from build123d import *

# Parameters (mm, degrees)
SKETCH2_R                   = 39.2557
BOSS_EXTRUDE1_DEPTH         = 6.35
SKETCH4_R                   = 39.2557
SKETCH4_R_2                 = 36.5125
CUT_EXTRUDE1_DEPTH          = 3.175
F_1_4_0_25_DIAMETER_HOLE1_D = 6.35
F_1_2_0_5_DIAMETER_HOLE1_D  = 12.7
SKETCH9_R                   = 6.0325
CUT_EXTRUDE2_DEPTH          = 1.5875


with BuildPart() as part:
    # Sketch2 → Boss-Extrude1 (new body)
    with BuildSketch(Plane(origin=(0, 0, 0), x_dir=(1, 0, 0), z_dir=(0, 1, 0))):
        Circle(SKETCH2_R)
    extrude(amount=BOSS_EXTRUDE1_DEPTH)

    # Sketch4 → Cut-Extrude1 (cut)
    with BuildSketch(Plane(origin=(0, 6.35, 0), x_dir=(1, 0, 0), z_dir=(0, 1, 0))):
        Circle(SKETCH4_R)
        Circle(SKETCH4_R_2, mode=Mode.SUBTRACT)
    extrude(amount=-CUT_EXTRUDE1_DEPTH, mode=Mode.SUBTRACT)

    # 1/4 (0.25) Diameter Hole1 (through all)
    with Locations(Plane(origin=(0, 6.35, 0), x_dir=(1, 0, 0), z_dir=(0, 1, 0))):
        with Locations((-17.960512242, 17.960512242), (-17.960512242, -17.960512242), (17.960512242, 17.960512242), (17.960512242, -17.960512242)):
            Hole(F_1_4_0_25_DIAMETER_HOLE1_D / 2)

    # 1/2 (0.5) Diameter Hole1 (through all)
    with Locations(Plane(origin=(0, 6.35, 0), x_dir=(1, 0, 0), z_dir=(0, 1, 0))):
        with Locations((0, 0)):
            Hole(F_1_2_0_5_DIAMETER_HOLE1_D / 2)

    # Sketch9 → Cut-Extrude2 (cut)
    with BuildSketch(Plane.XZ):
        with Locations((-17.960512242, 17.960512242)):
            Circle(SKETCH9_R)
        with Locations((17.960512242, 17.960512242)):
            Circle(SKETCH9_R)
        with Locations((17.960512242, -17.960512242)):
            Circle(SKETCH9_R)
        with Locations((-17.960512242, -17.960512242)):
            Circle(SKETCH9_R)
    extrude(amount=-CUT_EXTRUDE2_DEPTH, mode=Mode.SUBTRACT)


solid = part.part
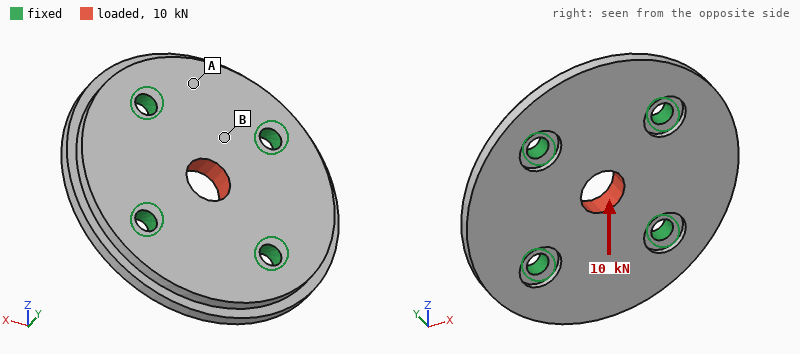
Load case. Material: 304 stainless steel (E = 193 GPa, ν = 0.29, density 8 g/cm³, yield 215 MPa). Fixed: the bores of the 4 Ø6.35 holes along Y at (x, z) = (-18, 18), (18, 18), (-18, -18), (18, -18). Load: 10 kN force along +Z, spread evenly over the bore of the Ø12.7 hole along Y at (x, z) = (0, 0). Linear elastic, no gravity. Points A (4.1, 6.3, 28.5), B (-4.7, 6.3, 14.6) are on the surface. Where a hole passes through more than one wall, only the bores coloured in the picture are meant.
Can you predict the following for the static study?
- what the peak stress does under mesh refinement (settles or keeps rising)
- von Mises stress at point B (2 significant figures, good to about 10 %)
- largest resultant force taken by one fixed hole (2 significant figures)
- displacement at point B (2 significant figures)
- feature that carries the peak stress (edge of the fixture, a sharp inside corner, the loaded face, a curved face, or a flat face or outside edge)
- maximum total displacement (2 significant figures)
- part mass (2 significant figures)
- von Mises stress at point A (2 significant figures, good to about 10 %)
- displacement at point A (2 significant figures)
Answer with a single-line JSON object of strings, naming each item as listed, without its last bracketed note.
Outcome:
{"what the peak stress does under mesh refinement": "keeps rising", "von Mises stress at point B": "24 MPa", "largest resultant force taken by one fixed hole": "2.6 kN", "displacement at point B": "2.3 µm", "feature that carries the peak stress": "edge of the fixture", "maximum total displacement": "4.1 µm", "part mass": "210 g", "von Mises stress at point A": "9.8 MPa", "displacement at point A": "1.6 µm"}
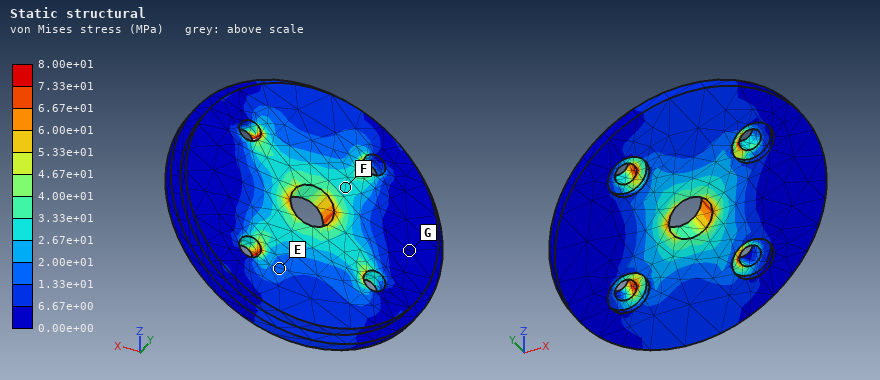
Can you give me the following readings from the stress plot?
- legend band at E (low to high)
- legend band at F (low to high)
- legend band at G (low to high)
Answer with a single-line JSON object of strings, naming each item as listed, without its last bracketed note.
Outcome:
{"legend band at E": "1.33e+01 to 2.00e+01 MPa", "legend band at F": "2.67e+01 to 3.33e+01 MPa", "legend band at G": "0.00e+00 to 6.67e+00 MPa"}
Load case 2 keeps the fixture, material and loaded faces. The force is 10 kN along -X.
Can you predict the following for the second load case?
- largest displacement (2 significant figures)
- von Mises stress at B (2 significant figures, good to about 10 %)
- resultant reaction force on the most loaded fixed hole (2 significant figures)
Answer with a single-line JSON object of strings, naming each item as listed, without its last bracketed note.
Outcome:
{"largest displacement": "4.1 µm", "von Mises stress at B": "20 MPa", "resultant reaction force on the most loaded fixed hole": "2.6 kN"}
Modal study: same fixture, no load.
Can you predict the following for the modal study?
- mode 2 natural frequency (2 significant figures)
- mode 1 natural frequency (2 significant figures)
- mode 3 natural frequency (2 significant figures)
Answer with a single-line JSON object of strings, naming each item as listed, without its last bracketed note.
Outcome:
{"mode 2 natural frequency": "11 kHz", "mode 1 natural frequency": "10 kHz", "mode 3 natural frequency": "11 kHz"}
